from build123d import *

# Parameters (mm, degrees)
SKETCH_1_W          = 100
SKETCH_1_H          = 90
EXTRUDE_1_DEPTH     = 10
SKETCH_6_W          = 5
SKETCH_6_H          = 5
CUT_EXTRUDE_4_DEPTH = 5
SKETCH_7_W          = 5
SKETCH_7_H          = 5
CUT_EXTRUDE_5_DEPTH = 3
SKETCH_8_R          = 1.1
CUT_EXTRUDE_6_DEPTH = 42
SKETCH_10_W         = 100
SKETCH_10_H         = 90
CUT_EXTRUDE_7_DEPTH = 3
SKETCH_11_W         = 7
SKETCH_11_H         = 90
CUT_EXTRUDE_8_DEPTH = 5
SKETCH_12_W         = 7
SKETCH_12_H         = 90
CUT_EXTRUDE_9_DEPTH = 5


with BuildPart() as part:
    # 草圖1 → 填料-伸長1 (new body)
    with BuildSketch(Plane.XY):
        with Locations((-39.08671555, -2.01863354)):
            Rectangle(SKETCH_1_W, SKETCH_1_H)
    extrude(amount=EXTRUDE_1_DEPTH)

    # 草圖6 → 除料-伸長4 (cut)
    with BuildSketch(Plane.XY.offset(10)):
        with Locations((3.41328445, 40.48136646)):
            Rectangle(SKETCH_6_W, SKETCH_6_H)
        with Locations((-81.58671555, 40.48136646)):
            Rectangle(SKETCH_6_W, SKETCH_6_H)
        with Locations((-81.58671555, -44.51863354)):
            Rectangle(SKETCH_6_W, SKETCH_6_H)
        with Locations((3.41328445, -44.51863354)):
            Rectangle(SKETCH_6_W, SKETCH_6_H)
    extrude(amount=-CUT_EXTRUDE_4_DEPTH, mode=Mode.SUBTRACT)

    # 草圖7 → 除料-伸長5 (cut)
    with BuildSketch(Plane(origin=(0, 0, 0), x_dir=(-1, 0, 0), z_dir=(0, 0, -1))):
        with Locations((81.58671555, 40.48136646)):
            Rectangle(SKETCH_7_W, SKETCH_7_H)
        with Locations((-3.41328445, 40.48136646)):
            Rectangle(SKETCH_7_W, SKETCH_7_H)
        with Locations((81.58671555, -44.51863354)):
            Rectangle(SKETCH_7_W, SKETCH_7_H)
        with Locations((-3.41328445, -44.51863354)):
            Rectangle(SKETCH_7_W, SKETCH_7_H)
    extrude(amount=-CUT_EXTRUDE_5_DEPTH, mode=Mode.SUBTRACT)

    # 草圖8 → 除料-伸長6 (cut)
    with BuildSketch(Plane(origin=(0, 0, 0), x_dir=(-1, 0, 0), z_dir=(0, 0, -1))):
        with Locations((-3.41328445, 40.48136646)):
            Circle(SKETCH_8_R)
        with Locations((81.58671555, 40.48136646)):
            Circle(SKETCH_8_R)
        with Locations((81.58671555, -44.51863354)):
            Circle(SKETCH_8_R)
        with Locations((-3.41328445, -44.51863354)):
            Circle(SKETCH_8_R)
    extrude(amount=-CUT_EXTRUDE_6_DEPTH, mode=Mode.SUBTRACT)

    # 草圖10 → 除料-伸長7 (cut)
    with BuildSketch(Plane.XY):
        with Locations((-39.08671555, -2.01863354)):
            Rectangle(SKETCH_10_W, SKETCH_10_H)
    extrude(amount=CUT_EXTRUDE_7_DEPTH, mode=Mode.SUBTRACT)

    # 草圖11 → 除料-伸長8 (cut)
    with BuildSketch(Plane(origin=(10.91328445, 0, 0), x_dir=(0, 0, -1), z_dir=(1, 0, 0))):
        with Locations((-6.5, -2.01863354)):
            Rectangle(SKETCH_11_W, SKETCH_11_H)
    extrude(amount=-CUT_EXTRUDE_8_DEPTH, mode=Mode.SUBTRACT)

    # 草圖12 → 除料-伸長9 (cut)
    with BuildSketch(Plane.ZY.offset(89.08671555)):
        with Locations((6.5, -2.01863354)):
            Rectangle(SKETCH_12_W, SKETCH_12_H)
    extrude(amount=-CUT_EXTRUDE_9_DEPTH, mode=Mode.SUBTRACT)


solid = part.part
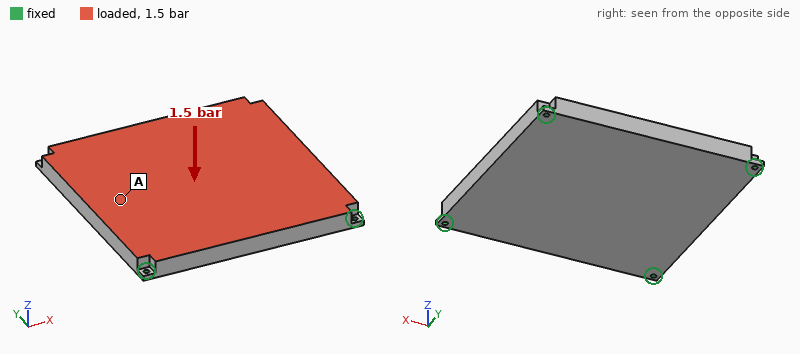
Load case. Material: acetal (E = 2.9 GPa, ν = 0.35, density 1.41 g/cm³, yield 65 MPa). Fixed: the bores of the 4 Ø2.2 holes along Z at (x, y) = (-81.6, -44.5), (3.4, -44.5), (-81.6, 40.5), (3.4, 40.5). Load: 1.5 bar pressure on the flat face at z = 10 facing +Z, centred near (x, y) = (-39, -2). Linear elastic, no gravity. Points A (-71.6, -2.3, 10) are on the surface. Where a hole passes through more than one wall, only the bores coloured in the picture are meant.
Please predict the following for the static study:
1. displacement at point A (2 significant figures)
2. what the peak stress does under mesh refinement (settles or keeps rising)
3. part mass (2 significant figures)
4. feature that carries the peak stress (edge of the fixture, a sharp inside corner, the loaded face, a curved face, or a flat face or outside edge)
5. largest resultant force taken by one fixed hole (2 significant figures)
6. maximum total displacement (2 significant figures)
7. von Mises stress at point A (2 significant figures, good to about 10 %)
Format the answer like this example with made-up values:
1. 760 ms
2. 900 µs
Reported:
1. 1.1 mm
2. keeps rising
3. 79 g
4. edge of the fixture
5. 660 N
6. 1.4 mm
7. 13 MPa
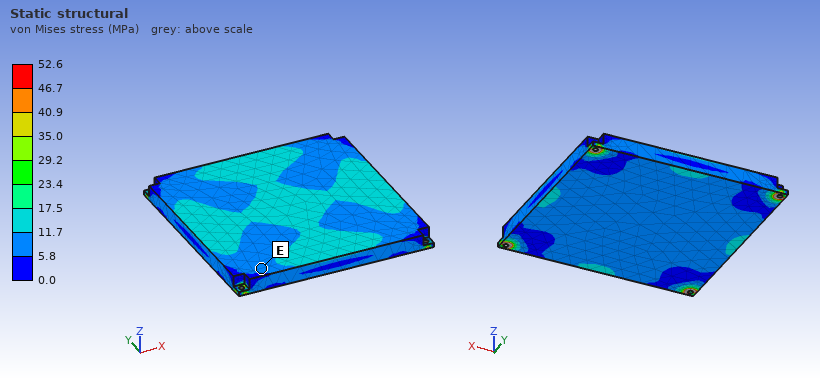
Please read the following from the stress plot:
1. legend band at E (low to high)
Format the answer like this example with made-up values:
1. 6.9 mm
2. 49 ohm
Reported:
1. 5.8 to 11.7 MPa
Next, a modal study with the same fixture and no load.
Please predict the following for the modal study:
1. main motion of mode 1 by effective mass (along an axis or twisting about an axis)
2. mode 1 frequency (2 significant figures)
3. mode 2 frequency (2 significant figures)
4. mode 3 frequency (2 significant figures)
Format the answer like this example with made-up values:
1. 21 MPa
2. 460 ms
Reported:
1. along Z
2. 600 Hz
3. 1100 Hz
4. 1100 Hz
